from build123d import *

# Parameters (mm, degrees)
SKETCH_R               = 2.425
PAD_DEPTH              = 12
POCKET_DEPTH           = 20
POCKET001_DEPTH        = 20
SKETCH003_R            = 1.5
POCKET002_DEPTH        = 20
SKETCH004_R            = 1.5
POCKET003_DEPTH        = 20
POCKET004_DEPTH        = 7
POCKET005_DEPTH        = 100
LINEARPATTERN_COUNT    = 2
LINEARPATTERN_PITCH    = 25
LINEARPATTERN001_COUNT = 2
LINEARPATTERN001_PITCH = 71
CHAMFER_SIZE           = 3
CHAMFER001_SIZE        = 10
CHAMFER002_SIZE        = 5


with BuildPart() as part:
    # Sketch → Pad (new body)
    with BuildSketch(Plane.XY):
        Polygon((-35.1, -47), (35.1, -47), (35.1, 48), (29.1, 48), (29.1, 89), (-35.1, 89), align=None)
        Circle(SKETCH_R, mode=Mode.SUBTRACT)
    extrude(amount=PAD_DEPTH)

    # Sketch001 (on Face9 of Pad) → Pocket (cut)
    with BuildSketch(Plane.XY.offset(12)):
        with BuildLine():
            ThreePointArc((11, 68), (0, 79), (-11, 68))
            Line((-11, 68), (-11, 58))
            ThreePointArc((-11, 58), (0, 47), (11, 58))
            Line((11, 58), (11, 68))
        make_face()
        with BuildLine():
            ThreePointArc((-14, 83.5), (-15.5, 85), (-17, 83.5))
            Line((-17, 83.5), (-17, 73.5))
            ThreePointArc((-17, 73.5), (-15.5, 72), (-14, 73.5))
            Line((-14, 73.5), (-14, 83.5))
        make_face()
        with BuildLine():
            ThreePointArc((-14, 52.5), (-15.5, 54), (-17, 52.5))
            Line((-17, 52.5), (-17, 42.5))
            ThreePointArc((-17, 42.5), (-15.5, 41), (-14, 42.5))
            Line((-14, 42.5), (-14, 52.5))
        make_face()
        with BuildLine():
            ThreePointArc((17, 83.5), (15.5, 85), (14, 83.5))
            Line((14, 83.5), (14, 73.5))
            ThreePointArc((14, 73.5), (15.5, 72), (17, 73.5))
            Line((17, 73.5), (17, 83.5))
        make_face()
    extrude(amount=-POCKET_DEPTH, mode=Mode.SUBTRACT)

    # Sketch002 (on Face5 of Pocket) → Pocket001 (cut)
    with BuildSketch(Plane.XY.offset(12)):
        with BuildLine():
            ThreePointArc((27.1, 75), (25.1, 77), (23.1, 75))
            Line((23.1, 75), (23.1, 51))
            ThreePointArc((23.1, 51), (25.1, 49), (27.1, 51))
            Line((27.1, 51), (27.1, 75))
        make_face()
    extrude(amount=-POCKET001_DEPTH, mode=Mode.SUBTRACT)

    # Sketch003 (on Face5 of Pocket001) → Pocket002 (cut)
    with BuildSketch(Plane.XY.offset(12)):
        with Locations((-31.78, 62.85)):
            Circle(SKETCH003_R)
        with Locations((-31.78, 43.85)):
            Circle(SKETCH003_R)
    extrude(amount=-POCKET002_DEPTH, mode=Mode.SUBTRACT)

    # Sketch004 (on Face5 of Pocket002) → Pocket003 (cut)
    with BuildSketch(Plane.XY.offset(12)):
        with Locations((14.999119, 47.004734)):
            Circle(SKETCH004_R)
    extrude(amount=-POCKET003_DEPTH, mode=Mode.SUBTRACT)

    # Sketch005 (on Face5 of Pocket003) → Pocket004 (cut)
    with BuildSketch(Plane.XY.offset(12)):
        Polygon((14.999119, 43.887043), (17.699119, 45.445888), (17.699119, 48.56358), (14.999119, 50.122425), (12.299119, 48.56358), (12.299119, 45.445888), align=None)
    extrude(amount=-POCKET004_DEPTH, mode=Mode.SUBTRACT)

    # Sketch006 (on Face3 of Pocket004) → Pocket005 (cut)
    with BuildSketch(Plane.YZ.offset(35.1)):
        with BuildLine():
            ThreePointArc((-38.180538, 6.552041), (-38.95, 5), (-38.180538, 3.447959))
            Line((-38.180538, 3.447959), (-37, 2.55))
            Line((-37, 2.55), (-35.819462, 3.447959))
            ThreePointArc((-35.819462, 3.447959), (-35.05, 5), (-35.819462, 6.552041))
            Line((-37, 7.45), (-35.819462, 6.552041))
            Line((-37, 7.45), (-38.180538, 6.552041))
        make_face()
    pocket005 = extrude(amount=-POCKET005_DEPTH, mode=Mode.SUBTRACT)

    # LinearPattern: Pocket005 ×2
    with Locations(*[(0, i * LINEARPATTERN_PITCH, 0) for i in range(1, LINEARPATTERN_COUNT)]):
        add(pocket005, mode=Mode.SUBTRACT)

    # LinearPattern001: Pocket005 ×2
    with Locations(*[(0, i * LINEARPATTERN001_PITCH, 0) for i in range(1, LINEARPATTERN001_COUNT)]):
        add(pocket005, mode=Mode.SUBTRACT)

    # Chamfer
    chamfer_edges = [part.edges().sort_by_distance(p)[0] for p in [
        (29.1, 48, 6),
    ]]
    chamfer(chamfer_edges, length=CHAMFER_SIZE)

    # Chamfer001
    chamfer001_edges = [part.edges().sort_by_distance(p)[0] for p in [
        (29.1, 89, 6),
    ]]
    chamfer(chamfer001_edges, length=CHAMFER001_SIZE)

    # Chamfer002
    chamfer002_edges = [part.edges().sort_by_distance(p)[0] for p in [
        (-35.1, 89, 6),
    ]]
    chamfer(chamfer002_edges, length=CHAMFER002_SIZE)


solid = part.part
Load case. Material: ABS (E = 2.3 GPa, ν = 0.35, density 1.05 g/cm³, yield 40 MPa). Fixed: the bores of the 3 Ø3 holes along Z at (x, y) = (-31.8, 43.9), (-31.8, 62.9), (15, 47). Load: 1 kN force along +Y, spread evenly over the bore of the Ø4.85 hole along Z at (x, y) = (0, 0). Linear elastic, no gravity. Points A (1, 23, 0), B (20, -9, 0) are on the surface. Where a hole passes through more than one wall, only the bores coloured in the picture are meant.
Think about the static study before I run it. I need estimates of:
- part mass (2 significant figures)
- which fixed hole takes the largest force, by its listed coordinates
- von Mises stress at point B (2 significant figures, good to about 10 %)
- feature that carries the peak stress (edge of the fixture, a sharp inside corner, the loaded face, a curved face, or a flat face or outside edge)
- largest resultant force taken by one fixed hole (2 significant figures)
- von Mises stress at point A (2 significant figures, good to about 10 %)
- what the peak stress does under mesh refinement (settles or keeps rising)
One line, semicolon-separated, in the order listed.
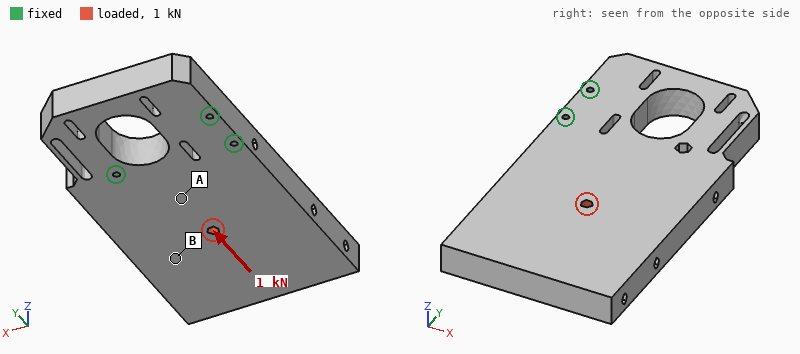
100 g; (15, 47); 0.81 MPa; edge of the fixture; 620 N; 2.0 MPa; keeps rising
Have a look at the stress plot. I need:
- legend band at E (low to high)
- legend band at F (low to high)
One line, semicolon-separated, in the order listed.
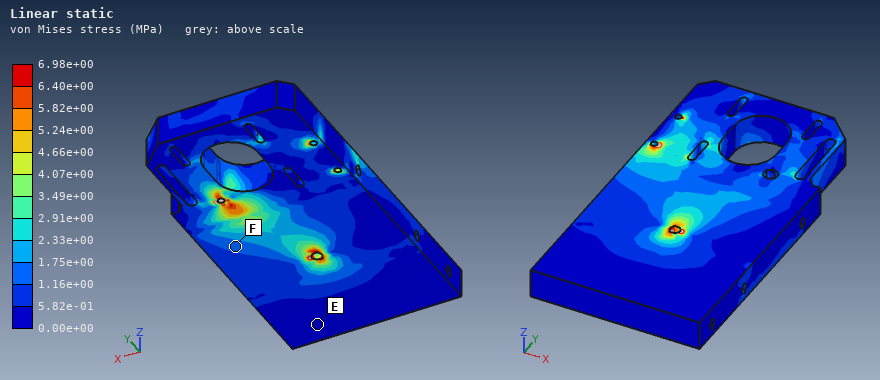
0.00e+00 to 5.82e-01 MPa; 1.16e+00 to 1.75e+00 MPa
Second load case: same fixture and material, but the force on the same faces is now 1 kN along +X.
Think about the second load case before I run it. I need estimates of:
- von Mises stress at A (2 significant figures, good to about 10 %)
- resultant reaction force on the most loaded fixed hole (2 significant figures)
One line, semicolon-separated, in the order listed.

3.8 MPa; 1.0 kN
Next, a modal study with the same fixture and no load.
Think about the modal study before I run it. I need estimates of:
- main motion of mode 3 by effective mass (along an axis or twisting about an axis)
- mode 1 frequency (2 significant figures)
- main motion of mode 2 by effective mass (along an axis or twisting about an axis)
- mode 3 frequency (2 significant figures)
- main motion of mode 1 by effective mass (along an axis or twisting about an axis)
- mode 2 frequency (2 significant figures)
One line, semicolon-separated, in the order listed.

along X; 240 Hz; twisting about Y; 1000 Hz; along Z; 820 Hz
